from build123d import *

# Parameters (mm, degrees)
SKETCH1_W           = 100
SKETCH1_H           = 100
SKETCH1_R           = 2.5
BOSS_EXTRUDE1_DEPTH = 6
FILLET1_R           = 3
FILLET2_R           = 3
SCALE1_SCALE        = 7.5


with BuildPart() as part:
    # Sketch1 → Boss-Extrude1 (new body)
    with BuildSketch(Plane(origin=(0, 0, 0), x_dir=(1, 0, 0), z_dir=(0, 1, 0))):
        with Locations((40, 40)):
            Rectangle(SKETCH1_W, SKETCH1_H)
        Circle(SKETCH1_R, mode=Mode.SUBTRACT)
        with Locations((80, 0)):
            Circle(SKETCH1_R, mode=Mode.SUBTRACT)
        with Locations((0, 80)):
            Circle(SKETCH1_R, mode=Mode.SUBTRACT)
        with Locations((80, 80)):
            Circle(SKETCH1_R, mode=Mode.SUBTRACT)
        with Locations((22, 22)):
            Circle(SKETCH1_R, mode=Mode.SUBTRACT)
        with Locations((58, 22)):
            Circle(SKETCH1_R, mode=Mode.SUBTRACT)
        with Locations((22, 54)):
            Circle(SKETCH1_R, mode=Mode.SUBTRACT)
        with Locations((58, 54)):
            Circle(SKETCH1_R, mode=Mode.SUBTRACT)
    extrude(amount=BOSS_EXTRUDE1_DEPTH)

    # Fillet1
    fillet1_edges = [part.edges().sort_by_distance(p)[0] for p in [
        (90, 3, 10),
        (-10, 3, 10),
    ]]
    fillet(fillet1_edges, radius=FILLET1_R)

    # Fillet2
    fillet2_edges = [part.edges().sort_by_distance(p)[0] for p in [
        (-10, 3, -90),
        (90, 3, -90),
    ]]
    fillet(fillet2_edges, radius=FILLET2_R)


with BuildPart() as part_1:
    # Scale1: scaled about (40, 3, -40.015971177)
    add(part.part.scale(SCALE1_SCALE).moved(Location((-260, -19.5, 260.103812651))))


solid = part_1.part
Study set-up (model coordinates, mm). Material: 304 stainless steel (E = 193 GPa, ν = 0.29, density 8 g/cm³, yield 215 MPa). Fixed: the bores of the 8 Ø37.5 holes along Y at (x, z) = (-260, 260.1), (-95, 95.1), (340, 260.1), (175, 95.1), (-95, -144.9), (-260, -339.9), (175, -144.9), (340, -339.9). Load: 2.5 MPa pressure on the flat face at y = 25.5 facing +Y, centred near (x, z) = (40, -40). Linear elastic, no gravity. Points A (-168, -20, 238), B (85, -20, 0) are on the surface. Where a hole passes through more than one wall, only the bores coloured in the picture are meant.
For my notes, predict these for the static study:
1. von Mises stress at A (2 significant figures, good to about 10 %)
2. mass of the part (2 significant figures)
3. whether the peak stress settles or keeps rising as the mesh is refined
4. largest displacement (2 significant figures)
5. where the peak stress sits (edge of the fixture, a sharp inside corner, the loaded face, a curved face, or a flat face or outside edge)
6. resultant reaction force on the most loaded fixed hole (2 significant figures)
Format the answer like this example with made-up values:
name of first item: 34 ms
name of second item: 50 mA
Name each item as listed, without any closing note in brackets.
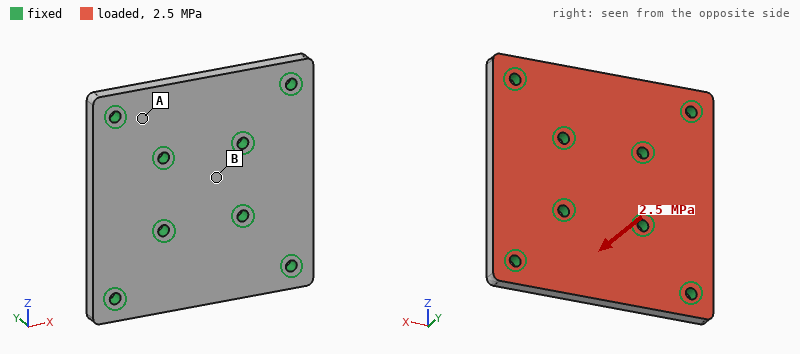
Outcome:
von Mises stress at A: 56 MPa
mass of the part: 200 kg
whether the peak stress settles or keeps rising as the mesh is refined: keeps rising
largest displacement: 0.37 mm
where the peak stress sits: edge of the fixture
resultant reaction force on the most loaded fixed hole: 210 kN
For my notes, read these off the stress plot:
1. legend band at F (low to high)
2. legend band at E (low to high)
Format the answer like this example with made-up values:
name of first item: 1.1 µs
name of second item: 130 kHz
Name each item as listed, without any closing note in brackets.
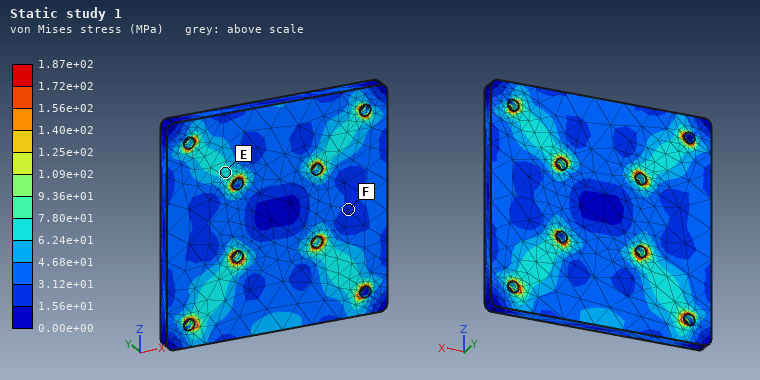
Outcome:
legend band at F: 1.56e+01 to 3.12e+01 MPa
legend band at E: 6.24e+01 to 7.80e+01 MPa
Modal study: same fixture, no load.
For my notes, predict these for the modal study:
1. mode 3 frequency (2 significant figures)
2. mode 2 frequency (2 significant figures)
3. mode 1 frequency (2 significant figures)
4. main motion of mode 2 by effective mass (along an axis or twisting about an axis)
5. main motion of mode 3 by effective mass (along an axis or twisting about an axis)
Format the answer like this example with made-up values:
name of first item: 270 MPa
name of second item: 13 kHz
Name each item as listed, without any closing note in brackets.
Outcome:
mode 3 frequency: 970 Hz
mode 2 frequency: 930 Hz
mode 1 frequency: 840 Hz
main motion of mode 2 by effective mass: twisting about X
main motion of mode 3 by effective mass: twisting about Z
